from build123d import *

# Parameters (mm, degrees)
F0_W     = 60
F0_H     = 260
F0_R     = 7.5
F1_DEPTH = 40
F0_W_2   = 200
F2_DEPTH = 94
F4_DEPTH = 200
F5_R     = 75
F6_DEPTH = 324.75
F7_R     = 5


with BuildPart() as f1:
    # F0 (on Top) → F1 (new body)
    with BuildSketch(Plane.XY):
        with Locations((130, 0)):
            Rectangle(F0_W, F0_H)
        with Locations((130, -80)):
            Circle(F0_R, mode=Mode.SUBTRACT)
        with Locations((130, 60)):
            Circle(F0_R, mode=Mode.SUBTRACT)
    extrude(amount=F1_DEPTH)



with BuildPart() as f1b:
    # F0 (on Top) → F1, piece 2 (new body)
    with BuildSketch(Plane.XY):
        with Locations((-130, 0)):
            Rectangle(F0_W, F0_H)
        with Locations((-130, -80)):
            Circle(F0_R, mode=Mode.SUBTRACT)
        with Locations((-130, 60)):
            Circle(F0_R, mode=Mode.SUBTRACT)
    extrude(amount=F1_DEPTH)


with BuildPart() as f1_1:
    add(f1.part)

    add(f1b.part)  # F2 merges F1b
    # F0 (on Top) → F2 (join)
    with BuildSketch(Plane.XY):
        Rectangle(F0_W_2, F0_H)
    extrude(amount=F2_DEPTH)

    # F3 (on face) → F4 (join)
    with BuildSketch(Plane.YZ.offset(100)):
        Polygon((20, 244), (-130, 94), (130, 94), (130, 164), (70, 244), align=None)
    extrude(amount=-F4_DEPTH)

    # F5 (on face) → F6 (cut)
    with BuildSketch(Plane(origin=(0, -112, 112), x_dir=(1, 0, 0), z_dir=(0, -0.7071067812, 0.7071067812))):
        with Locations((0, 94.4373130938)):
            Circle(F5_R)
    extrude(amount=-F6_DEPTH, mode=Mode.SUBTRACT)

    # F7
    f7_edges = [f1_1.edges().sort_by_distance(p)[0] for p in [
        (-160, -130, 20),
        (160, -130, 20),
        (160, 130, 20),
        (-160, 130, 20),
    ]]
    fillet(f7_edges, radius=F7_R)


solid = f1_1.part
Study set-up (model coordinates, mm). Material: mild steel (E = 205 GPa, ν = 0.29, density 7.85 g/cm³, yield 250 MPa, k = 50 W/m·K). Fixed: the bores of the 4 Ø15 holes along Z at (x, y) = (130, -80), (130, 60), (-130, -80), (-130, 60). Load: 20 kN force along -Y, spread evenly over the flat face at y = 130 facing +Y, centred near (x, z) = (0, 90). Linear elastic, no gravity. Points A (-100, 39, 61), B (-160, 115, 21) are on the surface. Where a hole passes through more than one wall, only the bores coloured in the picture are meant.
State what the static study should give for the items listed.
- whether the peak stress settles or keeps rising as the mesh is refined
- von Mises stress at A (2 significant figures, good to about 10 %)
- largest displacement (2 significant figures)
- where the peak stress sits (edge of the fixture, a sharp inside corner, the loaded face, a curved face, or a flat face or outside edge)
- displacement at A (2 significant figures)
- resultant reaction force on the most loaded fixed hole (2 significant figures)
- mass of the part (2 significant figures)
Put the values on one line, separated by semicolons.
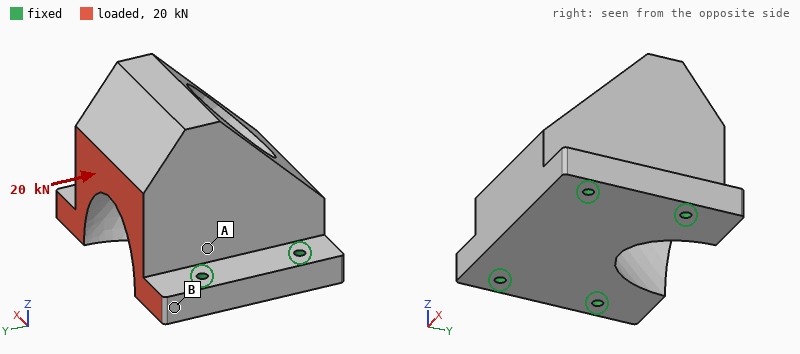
keeps rising; 3.2 MPa; 8.9 µm; edge of the fixture; 2.5 µm; 7.5 kN; 57 kg
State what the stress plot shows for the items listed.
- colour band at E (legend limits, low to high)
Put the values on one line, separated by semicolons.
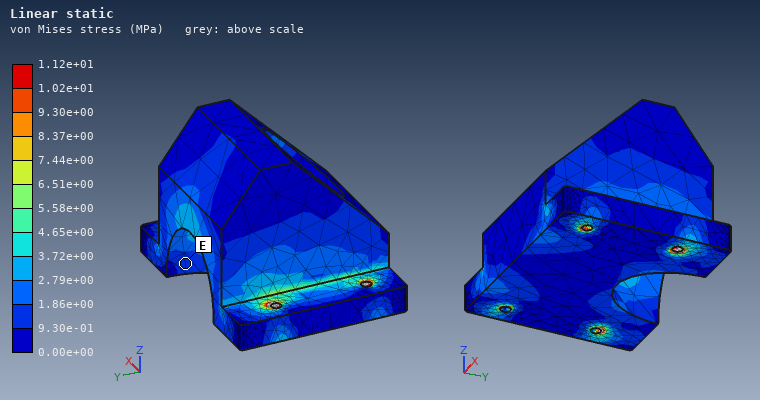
9.30e-01 to 1.86e+00 MPa
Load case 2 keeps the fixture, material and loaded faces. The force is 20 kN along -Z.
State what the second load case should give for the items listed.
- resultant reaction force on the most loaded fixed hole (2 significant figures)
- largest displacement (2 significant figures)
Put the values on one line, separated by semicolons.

14 kN; 13 µm
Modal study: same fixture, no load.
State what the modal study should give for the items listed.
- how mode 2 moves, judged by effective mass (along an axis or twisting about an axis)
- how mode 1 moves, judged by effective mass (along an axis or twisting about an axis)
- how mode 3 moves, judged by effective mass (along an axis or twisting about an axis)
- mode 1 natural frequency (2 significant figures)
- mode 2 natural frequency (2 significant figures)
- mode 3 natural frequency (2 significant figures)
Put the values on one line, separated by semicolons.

along X; along Y; along Z; 1200 Hz; 1400 Hz; 2200 Hz
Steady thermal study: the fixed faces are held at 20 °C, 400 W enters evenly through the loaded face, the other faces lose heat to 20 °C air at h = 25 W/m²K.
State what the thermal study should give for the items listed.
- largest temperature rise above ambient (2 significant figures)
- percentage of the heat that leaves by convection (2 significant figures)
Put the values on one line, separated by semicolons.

66 K; 45 %
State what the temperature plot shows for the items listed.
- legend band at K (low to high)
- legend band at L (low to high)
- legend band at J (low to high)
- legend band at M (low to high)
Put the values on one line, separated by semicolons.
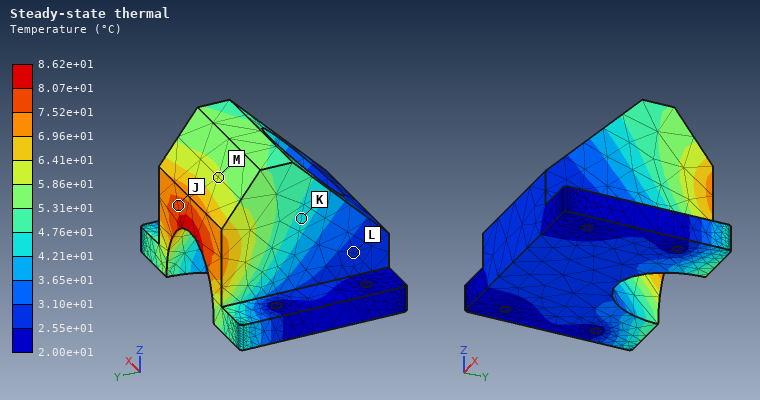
4.21e+01 to 4.76e+01 °C; 2.55e+01 to 3.10e+01 °C; 7.52e+01 to 8.07e+01 °C; 5.86e+01 to 6.41e+01 °C
